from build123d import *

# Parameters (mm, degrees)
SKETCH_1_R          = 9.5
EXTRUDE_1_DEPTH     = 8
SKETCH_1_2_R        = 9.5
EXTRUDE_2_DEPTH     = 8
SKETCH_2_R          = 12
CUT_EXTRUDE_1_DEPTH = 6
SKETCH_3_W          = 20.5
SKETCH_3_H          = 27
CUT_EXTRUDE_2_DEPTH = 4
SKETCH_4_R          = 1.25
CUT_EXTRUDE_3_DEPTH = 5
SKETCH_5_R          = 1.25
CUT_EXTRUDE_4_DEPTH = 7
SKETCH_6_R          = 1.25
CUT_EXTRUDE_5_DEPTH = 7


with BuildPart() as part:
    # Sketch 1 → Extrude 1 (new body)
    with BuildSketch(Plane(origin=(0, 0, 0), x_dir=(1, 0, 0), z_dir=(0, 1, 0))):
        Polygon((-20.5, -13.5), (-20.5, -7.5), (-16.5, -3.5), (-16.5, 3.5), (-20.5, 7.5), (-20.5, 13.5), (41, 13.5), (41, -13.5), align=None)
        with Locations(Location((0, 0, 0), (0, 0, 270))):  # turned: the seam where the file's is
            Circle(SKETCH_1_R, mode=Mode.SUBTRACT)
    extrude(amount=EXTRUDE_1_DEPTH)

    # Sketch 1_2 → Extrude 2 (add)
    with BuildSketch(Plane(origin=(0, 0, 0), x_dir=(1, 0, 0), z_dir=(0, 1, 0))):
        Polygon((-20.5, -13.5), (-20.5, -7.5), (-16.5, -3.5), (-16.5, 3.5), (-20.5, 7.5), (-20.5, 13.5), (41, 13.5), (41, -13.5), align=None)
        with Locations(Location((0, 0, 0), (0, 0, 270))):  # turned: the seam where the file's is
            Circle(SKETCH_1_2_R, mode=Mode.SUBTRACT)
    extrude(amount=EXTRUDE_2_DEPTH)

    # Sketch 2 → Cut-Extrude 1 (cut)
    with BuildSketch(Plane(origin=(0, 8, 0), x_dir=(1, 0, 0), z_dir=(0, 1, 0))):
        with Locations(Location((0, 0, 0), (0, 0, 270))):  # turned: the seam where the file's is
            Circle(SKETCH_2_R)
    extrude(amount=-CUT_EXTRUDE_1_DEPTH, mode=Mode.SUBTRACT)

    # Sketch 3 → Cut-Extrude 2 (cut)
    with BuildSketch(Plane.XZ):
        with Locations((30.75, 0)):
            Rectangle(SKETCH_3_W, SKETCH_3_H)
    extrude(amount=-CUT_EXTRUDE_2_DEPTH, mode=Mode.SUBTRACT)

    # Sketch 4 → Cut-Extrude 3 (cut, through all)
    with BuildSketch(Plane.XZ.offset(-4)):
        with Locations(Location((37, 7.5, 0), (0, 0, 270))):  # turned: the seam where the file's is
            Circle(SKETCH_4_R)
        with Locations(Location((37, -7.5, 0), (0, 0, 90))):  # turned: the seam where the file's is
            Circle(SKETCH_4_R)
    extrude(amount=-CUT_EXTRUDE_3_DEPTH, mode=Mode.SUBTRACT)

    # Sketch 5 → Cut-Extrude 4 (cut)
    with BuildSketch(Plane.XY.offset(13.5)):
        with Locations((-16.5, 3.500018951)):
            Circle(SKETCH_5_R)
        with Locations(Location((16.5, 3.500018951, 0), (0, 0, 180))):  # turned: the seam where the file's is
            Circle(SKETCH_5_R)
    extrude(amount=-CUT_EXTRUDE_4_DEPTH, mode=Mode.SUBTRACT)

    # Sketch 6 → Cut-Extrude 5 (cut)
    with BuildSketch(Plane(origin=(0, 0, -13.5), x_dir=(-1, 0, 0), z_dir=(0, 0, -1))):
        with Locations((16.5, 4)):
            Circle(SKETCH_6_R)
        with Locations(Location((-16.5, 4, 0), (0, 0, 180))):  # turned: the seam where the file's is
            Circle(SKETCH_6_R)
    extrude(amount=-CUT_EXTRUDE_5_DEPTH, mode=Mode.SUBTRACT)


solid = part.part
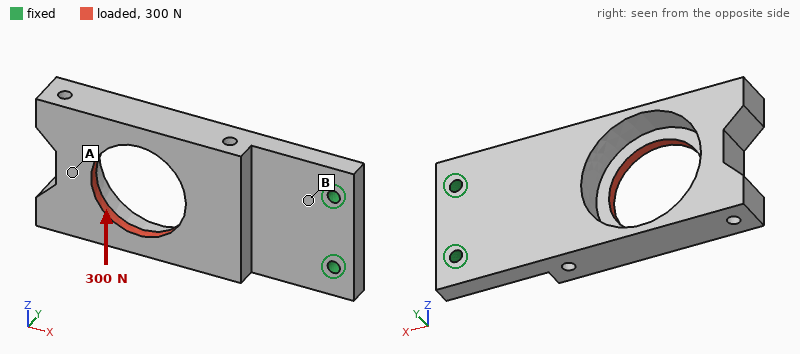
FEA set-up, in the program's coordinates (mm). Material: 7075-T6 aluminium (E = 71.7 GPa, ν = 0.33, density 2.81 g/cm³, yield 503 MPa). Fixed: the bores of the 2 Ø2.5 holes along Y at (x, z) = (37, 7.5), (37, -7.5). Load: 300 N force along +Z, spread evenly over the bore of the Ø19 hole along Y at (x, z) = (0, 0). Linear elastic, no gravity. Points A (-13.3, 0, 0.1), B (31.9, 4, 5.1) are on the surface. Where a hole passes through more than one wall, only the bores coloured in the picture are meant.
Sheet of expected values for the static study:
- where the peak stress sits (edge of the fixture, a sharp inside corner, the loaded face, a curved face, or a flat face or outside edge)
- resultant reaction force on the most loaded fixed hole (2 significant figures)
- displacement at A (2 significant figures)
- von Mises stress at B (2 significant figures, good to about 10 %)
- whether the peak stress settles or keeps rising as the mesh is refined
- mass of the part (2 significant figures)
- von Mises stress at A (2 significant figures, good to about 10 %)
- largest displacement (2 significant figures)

edge of the fixture
690 N
47 µm
22 MPa
keeps rising
20 g
6.5 MPa
53 µm
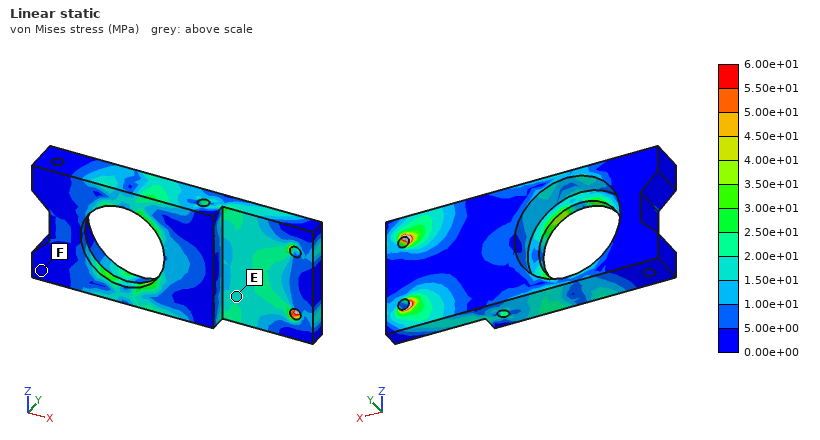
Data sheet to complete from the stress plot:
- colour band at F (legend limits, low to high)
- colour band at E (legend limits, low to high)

0.00e+00 to 5.00e+00 MPa
1.50e+01 to 2.00e+01 MPa
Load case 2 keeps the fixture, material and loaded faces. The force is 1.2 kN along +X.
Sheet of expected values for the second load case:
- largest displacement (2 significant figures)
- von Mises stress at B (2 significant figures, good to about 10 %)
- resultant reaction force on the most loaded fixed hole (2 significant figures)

0.57 mm
90 MPa
600 N
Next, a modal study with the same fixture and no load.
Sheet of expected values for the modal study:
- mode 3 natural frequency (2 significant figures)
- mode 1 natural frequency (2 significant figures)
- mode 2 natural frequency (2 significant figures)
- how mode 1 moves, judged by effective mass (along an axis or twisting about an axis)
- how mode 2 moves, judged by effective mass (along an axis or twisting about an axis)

4200 Hz
980 Hz
3600 Hz
along Y
along Z
